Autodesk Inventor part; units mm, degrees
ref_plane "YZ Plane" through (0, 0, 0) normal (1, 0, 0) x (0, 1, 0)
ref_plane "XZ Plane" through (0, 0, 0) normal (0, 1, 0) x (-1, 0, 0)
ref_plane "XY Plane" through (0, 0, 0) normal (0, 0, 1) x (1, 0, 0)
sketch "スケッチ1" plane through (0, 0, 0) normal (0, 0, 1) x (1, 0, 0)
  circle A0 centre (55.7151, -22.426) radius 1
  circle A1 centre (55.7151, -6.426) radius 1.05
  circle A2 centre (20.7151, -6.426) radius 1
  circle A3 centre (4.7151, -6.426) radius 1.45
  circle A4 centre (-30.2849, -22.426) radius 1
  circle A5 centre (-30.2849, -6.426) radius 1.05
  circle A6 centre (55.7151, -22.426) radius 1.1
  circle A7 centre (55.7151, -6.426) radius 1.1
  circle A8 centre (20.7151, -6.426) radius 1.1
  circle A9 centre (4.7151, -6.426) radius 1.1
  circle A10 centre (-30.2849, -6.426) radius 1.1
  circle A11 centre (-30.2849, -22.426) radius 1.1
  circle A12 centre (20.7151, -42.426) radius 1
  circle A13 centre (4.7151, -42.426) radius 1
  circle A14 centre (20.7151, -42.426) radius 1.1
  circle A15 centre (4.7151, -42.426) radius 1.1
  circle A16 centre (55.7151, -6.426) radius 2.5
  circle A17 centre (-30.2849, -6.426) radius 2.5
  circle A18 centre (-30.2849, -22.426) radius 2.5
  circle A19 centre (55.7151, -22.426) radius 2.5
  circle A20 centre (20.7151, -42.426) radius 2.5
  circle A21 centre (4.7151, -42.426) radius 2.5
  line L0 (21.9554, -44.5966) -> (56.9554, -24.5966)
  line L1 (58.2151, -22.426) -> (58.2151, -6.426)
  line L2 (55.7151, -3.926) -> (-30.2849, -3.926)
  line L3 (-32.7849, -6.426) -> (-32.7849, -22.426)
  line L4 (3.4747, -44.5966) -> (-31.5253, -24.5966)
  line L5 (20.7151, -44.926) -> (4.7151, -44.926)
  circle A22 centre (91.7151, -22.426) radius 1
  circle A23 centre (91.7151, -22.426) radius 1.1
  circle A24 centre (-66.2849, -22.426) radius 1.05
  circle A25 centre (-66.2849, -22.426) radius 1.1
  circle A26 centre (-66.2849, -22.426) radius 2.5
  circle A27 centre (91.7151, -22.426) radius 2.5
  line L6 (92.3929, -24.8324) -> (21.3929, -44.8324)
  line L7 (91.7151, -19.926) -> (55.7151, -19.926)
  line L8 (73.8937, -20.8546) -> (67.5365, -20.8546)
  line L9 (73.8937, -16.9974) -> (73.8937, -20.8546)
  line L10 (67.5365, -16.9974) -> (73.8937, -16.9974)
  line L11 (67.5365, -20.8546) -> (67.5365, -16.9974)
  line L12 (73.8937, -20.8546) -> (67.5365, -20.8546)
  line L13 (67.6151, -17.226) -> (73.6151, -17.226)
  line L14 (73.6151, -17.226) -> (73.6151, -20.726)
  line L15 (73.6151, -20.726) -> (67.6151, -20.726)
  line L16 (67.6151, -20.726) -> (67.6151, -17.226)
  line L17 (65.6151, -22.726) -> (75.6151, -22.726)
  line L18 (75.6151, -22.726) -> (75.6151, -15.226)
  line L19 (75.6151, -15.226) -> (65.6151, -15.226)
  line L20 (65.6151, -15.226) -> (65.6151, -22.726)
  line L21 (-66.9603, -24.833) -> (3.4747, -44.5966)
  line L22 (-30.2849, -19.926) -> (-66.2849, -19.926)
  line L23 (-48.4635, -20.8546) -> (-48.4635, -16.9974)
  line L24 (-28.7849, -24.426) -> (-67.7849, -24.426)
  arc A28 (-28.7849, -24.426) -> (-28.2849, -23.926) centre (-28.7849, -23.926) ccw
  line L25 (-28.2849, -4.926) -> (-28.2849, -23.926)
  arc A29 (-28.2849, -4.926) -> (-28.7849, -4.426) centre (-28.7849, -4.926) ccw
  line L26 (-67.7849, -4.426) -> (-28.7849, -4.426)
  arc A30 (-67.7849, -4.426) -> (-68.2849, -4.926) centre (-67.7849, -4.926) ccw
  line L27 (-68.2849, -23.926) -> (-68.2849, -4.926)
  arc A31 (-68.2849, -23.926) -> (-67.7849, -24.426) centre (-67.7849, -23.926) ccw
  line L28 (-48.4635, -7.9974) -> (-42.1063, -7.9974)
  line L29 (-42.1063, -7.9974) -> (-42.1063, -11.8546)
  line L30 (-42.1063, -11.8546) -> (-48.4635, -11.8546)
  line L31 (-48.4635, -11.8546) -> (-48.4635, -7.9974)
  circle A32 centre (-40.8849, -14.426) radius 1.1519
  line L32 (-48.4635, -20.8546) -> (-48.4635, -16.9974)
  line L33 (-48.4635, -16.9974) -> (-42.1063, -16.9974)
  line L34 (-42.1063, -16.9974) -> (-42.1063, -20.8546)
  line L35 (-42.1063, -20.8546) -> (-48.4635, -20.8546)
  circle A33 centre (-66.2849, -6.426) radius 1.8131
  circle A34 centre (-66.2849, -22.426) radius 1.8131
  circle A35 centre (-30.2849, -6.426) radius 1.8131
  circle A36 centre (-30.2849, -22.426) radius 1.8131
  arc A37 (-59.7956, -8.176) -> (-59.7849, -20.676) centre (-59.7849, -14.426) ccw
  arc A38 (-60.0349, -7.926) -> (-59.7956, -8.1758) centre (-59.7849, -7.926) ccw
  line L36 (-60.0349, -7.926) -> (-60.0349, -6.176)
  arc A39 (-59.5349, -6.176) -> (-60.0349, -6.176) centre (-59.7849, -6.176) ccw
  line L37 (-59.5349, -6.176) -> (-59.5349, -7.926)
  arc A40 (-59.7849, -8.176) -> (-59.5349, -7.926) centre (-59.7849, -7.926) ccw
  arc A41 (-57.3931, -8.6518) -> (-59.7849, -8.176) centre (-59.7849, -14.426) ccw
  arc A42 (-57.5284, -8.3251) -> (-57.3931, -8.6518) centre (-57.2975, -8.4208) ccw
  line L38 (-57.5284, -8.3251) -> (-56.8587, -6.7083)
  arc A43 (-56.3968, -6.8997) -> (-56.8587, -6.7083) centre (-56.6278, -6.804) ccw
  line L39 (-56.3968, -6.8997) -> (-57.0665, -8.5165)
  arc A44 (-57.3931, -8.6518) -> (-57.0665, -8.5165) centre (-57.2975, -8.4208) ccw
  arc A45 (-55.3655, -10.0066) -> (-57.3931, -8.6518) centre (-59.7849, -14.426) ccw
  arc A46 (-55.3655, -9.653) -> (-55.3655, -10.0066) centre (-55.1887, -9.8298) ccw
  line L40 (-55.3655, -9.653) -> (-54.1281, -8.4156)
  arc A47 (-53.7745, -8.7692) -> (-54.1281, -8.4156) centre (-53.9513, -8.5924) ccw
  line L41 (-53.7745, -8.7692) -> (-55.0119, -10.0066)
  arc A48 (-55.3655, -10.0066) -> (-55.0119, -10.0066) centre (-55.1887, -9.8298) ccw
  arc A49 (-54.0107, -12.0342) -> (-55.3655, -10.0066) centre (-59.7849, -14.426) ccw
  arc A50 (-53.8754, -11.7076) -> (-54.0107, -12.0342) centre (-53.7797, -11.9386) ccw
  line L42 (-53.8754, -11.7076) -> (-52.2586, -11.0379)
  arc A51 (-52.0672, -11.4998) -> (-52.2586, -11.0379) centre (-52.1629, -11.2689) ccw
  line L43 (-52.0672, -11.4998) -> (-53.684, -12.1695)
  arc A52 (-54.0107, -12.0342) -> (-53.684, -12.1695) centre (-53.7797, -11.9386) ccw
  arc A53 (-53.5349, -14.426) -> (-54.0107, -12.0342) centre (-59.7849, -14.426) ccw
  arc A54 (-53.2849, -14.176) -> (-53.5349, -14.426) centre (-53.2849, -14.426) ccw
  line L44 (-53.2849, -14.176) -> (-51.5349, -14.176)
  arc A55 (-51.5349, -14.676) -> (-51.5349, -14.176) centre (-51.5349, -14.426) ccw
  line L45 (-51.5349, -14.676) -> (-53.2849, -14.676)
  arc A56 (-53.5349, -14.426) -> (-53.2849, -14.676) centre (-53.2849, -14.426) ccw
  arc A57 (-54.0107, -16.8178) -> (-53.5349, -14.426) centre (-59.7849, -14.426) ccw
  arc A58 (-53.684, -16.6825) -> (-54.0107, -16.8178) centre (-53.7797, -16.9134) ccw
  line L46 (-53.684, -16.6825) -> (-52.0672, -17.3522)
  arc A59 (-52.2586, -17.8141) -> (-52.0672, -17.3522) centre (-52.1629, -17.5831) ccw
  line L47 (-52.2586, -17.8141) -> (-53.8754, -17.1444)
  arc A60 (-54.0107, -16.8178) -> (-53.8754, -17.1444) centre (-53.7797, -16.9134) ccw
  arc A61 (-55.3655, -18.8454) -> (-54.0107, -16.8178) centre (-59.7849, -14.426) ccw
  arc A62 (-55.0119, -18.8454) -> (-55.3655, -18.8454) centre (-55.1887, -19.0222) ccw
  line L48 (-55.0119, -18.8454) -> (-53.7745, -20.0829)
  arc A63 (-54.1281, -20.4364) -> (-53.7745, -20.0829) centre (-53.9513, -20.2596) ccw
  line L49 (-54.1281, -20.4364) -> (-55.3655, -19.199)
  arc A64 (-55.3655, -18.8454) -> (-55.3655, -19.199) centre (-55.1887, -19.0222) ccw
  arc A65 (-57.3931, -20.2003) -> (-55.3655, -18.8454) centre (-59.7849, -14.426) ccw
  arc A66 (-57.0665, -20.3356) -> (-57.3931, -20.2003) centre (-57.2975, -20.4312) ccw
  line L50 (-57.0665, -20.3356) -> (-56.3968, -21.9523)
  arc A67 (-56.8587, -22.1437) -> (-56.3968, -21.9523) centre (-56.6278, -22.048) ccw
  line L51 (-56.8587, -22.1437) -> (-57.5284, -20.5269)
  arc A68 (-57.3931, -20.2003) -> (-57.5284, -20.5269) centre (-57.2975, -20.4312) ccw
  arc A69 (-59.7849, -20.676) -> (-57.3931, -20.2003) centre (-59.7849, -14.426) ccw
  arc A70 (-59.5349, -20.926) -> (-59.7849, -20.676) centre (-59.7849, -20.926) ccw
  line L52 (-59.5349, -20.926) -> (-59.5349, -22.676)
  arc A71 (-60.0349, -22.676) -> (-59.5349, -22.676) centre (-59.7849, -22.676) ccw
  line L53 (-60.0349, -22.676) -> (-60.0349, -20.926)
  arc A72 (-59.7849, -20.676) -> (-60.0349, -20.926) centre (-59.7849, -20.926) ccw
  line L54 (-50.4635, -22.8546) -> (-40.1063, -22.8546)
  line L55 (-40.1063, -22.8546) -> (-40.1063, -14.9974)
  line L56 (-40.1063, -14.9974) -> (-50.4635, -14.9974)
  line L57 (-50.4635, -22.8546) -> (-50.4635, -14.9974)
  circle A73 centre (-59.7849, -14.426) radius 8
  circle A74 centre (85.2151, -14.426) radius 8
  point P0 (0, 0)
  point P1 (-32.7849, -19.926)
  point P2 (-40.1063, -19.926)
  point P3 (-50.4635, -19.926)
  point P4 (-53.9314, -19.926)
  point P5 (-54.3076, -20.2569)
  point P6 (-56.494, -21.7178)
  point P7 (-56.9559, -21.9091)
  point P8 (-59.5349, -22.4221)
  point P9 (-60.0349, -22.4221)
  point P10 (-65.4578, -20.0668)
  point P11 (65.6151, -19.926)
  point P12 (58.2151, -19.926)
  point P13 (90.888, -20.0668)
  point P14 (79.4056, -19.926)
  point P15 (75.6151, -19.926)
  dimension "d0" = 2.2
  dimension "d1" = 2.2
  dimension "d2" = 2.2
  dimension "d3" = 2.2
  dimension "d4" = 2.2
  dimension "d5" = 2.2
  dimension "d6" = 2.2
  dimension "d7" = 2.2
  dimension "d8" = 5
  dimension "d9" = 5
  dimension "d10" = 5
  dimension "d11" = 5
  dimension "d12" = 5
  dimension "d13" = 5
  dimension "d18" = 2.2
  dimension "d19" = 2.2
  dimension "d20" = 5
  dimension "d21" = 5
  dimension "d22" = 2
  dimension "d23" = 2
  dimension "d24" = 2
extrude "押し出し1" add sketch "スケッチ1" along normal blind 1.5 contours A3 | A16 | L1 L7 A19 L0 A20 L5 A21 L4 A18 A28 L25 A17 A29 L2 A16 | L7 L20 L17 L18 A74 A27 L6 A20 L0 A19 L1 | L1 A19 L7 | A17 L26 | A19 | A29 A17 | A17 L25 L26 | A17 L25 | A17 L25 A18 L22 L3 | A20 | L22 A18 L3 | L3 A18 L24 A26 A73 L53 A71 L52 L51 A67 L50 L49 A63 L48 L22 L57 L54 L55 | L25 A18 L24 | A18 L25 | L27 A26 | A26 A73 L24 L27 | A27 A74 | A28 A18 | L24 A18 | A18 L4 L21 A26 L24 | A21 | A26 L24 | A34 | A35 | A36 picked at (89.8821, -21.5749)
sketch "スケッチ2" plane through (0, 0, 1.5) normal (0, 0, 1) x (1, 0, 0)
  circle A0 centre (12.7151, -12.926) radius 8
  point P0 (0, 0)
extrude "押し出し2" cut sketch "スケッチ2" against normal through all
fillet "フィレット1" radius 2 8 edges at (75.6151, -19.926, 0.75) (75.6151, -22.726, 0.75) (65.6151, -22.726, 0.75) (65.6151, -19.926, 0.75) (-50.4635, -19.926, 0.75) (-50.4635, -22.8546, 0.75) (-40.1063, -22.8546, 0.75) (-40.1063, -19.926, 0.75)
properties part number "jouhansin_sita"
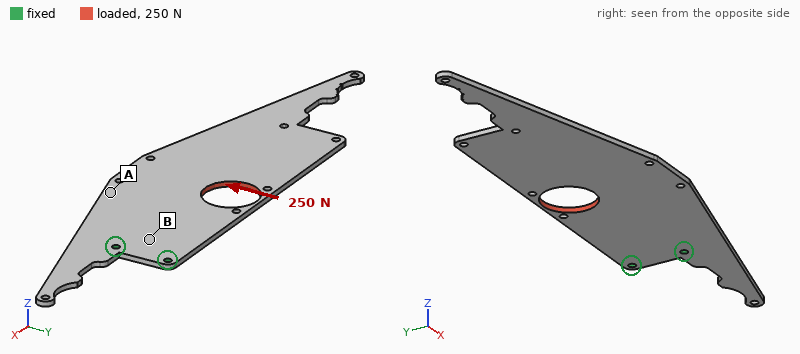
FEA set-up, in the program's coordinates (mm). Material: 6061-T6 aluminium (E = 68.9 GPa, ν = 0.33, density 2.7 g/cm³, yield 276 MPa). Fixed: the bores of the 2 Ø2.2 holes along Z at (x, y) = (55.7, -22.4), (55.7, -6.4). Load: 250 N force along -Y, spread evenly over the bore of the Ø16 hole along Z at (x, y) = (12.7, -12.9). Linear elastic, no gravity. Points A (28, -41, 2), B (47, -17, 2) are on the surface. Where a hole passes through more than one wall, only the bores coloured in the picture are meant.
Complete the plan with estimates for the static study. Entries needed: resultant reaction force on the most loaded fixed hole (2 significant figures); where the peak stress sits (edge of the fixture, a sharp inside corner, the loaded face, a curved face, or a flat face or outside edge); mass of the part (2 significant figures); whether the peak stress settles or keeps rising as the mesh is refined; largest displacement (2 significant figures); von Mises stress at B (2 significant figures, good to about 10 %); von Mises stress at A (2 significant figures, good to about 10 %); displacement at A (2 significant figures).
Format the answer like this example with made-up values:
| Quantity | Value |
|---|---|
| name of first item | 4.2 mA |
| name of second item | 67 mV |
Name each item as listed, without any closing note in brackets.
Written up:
| Quantity | Value |
|---|---|
| resultant reaction force on the most loaded fixed hole | 660 N |
| where the peak stress sits | edge of the fixture |
| mass of the part | 15 g |
| whether the peak stress settles or keeps rising as the mesh is refined | keeps rising |
| largest displacement | 0.19 mm |
| von Mises stress at B | 28 MPa |
| von Mises stress at A | 8.5 MPa |
| displacement at A | 0.050 mm |
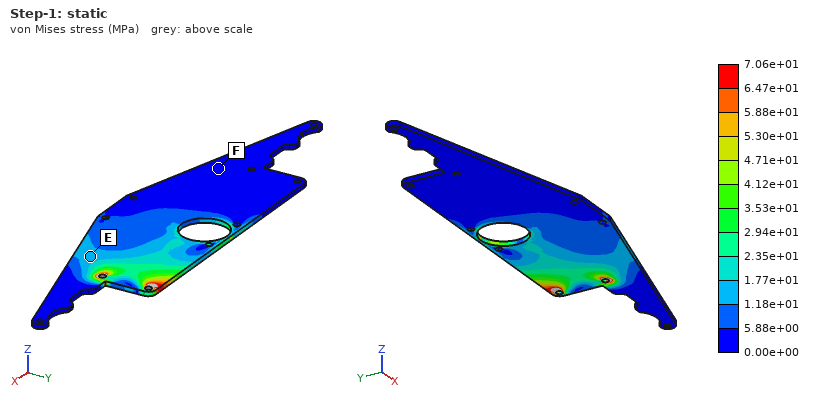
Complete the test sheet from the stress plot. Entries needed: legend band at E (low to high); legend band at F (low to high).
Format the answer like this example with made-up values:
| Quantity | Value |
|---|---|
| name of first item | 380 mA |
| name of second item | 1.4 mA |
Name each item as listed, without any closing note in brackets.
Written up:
| Quantity | Value |
|---|---|
| legend band at E | 1.18e+01 to 1.77e+01 MPa |
| legend band at F | 0.00e+00 to 5.88e+00 MPa |
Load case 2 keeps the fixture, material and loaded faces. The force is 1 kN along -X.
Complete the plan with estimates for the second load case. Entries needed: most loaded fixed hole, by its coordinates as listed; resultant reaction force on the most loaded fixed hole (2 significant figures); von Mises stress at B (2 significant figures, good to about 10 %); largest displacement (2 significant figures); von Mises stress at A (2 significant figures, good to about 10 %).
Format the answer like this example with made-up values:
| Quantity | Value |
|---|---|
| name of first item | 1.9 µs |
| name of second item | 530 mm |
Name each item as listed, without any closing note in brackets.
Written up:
| Quantity | Value |
|---|---|
| most loaded fixed hole, by its coordinates as listed | (55.7, -6.4) |
| resultant reaction force on the most loaded fixed hole | 600 N |
| von Mises stress at B | 20 MPa |
| largest displacement | 0.17 mm |
| von Mises stress at A | 12 MPa |
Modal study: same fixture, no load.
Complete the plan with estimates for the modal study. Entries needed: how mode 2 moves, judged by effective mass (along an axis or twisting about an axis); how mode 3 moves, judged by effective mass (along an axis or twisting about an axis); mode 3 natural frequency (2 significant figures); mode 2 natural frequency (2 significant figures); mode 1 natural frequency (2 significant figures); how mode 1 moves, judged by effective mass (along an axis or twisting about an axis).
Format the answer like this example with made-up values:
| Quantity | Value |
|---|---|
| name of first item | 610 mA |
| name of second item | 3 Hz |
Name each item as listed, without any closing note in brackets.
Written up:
| Quantity | Value |
|---|---|
| how mode 2 moves, judged by effective mass | along Z |
| how mode 3 moves, judged by effective mass | twisting about X |
| mode 3 natural frequency | 700 Hz |
| mode 2 natural frequency | 610 Hz |
| mode 1 natural frequency | 120 Hz |
| how mode 1 moves, judged by effective mass | along Z |
